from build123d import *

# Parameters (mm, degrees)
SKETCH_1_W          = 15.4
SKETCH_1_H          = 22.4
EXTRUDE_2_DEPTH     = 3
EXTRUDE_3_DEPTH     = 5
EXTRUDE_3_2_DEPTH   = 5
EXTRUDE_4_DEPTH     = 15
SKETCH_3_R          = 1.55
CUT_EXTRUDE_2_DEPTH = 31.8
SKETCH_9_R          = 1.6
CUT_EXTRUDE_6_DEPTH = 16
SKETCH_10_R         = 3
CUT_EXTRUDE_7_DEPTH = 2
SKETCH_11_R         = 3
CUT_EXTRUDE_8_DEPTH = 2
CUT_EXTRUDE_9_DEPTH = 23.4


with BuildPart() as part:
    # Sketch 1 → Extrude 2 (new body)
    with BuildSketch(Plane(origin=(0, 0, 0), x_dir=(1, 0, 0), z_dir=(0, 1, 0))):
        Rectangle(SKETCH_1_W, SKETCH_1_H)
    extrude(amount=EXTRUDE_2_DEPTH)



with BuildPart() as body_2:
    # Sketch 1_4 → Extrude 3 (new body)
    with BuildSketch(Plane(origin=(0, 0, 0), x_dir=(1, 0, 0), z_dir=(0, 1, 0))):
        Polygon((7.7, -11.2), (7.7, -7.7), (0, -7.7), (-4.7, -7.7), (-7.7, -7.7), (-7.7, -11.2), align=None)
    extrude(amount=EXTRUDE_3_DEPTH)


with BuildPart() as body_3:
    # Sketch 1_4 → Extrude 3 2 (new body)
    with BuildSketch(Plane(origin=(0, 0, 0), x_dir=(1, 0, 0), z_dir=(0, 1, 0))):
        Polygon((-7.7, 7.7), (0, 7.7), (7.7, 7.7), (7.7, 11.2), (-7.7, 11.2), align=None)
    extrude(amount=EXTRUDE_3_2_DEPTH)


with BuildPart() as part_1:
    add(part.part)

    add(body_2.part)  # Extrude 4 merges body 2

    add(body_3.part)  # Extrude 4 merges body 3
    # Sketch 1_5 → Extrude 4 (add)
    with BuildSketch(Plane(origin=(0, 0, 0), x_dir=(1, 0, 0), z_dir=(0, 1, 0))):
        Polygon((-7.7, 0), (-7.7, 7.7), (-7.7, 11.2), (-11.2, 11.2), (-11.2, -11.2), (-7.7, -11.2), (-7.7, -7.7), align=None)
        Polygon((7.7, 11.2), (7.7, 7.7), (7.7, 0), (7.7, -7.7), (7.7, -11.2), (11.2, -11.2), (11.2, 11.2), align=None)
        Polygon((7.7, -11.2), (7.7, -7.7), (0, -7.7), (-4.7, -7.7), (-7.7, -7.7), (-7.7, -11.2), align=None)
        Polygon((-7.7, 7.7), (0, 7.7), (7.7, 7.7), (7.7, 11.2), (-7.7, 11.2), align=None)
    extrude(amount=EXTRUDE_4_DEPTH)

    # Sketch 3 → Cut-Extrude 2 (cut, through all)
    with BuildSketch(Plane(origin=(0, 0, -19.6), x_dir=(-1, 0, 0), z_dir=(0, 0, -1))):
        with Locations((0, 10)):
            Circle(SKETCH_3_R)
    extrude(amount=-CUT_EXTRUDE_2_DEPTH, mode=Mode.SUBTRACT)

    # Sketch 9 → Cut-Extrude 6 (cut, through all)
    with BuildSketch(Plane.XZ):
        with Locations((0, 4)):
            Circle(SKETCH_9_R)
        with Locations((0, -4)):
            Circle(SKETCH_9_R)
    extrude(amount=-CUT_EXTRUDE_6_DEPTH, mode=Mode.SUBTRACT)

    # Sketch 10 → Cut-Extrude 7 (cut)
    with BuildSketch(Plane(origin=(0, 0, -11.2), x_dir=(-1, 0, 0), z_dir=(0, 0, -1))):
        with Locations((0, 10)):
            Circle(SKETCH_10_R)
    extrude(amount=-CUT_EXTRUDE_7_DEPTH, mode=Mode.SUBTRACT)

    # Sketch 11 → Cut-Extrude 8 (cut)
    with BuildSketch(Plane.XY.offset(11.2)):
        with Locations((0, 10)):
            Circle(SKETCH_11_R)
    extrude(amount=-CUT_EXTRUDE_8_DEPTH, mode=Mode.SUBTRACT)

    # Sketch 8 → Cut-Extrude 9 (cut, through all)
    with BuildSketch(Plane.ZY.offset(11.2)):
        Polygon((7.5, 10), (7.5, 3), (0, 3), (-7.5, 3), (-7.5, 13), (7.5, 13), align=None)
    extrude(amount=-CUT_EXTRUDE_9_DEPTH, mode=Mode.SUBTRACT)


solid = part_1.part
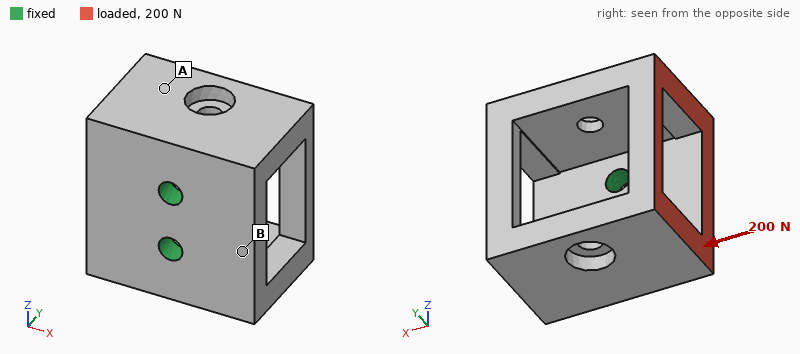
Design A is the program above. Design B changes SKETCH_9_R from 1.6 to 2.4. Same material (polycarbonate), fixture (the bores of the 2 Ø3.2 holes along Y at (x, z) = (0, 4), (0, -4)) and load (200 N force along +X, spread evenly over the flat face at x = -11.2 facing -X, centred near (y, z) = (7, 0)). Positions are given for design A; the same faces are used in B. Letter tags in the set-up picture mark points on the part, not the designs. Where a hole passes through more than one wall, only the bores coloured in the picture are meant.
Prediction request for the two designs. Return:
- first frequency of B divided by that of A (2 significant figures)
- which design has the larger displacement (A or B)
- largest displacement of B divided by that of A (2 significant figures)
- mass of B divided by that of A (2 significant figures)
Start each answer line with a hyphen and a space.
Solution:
- 1.1
- A
- 0.73
- 0.98
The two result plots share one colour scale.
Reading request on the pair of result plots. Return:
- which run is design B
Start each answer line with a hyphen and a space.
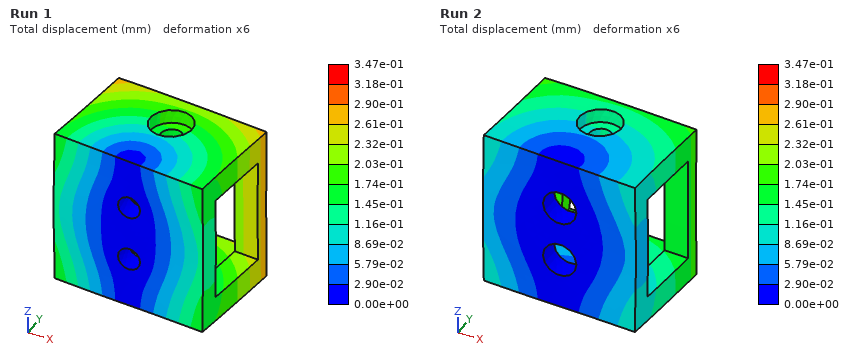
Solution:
- Run 2
